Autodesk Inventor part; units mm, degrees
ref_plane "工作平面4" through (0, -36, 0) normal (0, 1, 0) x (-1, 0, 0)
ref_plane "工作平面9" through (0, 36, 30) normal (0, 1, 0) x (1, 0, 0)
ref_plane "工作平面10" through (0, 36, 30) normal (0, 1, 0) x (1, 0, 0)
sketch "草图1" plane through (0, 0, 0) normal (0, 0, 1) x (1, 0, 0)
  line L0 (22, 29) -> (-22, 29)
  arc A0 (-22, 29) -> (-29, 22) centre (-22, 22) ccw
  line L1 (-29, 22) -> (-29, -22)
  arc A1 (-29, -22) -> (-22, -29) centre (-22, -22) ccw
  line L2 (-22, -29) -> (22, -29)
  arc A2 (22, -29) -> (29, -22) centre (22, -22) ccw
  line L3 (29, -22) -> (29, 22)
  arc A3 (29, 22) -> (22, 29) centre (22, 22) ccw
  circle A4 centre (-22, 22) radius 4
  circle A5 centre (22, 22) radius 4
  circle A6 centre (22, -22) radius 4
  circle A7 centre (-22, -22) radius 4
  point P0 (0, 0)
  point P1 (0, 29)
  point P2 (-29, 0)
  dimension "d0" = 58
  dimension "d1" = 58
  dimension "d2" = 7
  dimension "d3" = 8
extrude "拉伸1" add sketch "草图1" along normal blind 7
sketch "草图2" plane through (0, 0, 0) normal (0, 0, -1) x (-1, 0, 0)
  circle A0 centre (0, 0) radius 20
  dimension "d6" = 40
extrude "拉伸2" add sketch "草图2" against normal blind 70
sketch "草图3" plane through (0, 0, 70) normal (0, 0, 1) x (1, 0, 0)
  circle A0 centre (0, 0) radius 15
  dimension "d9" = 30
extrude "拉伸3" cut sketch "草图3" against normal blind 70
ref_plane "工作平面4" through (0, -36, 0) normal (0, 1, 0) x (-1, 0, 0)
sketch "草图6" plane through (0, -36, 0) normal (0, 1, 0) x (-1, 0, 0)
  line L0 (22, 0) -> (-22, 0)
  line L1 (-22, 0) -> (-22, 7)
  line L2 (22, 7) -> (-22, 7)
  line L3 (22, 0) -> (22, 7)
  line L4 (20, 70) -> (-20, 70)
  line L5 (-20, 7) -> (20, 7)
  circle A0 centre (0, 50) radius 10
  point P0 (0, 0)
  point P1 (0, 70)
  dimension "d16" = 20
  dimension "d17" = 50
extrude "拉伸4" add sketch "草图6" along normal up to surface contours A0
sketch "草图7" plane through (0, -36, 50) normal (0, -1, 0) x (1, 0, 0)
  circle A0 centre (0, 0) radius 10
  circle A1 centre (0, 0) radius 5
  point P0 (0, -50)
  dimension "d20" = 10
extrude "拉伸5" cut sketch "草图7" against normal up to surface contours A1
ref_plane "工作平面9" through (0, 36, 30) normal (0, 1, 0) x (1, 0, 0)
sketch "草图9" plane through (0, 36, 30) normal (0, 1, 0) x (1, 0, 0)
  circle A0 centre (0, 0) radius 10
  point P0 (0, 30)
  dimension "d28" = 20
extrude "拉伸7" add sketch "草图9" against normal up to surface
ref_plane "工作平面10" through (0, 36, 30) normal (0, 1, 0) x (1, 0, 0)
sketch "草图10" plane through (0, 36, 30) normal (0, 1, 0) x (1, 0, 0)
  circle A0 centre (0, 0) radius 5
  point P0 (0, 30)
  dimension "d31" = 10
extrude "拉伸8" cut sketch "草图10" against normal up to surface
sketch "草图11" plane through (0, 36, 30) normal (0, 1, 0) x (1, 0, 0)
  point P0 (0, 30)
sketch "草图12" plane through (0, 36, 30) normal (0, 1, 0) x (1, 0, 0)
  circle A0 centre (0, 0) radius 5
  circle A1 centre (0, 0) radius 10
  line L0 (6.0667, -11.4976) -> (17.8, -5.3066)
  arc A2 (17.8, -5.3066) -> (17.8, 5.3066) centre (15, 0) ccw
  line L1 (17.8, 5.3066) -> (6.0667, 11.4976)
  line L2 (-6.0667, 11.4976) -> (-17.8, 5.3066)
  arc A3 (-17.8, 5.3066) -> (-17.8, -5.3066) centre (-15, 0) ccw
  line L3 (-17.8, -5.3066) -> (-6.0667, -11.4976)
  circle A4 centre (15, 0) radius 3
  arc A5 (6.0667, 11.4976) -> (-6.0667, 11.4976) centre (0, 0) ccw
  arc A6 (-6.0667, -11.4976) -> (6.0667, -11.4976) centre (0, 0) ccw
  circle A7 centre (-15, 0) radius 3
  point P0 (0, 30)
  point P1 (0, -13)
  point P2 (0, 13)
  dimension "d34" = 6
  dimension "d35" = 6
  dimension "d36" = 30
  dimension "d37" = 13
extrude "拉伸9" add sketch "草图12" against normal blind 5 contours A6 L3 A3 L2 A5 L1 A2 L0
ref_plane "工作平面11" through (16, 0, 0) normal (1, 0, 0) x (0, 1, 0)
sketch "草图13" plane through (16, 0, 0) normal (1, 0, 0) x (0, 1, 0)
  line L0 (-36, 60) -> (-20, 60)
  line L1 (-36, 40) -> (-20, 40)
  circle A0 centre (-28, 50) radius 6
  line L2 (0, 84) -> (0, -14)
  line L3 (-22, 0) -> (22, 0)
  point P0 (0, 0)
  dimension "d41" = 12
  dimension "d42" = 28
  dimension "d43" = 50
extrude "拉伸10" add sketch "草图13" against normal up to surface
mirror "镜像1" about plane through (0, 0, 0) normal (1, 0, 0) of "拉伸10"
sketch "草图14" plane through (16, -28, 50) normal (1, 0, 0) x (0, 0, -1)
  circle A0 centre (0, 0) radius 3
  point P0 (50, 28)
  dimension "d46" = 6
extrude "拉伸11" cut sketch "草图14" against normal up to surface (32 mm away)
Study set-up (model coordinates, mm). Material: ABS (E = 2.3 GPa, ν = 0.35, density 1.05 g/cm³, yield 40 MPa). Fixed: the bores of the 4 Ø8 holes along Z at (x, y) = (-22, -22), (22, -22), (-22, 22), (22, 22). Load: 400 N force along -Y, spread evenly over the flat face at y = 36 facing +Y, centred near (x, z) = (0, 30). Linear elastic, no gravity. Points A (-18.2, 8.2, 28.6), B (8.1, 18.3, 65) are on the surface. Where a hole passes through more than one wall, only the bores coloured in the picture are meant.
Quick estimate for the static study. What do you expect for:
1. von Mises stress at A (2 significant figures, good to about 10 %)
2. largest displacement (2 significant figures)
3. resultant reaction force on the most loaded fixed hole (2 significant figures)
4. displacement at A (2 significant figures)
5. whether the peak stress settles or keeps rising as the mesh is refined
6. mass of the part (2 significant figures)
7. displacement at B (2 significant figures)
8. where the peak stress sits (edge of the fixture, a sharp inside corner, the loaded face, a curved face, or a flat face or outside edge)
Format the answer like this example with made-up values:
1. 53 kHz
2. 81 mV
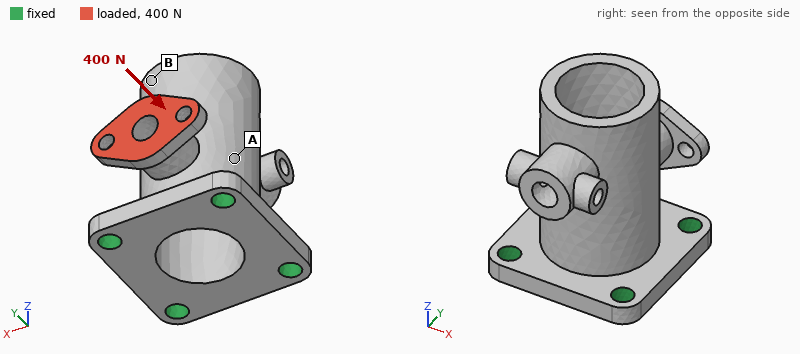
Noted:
1. 1.7 MPa
2. 0.28 mm
3. 180 N
4. 0.092 mm
5. keeps rising
6. 64 g
7. 0.21 mm
8. edge of the fixture
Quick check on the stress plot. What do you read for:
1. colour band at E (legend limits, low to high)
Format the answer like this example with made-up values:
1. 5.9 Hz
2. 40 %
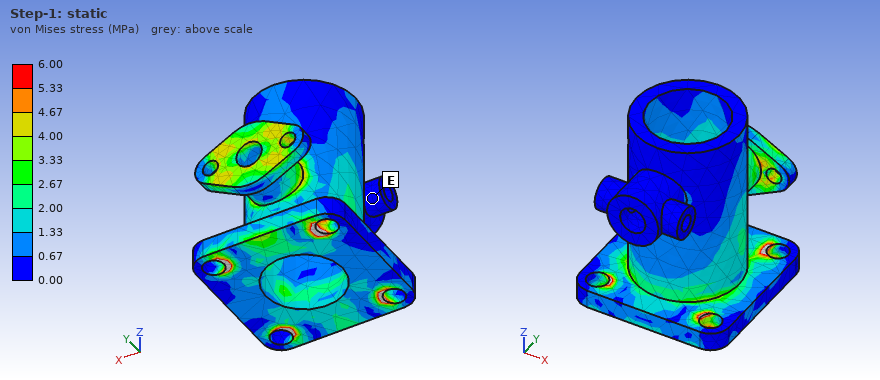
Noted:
1. 0.00 to 0.67 MPa
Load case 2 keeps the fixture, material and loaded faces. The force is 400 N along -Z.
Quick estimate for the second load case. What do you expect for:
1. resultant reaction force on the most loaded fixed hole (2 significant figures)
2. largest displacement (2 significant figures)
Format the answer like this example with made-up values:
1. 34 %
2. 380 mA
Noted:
1. 320 N
2. 0.54 mm
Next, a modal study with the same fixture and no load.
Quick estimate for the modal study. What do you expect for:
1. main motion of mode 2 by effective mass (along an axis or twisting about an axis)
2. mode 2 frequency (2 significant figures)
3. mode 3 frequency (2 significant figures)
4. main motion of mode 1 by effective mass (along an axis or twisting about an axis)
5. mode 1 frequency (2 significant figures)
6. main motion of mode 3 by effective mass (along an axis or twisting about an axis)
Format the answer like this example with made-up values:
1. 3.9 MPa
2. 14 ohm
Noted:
1. along X
2. 1000 Hz
3. 2100 Hz
4. along Y
5. 950 Hz
6. twisting about Z
